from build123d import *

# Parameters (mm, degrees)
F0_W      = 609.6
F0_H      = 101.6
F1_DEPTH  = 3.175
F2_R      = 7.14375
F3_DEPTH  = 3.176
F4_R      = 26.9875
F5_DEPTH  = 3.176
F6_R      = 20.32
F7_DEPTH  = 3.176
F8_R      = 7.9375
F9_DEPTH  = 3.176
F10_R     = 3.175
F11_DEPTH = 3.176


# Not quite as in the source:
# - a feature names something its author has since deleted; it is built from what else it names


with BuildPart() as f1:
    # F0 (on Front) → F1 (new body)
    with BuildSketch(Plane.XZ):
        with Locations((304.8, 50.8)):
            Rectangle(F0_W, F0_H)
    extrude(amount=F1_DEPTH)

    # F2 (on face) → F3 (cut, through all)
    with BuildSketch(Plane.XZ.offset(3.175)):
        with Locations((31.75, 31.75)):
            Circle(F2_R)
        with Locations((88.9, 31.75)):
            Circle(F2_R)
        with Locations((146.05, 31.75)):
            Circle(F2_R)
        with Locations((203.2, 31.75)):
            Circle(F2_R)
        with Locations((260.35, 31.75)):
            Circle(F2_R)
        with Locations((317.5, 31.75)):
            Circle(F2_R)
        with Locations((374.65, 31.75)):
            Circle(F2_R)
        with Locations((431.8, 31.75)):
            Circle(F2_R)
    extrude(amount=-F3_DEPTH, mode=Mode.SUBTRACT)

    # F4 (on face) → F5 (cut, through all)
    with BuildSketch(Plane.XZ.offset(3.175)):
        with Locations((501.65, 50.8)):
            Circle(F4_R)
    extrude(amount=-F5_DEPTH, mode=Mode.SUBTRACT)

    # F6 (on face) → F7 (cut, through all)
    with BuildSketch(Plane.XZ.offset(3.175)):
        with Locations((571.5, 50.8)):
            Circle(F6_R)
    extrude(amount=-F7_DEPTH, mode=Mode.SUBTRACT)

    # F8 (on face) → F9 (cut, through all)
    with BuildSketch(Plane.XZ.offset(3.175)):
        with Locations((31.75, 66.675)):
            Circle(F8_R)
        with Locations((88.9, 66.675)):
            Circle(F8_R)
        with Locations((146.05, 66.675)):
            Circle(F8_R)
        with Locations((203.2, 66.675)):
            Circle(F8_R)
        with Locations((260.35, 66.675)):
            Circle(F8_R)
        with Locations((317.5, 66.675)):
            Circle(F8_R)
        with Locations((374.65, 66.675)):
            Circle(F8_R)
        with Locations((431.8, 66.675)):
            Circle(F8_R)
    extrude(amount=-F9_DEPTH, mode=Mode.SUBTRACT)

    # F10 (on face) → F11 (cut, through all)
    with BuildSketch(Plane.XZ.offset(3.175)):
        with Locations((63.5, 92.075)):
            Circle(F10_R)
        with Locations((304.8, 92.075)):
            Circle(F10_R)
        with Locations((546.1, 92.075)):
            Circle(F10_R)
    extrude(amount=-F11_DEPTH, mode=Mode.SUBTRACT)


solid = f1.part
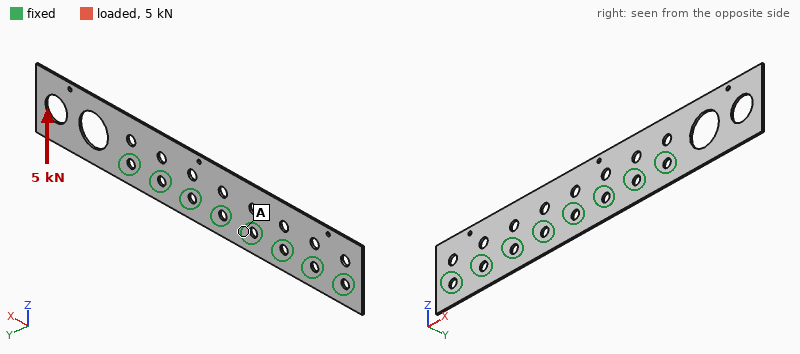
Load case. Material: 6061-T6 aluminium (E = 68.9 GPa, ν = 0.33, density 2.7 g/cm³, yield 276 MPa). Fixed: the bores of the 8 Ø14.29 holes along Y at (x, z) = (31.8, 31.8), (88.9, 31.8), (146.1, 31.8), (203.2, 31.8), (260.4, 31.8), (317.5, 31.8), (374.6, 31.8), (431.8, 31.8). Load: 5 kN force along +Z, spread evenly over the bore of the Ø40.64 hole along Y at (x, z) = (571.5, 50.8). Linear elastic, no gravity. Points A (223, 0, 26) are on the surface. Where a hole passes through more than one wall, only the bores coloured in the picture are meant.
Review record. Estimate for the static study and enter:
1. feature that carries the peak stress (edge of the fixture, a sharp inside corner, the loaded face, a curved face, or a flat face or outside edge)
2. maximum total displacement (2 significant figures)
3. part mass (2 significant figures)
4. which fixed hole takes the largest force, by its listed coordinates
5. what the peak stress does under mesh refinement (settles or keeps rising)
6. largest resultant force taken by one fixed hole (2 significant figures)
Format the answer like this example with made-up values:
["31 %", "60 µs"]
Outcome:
["edge of the fixture", "1.1 mm", "470 g", "(431.8, 31.8)", "keeps rising", "11 kN"]
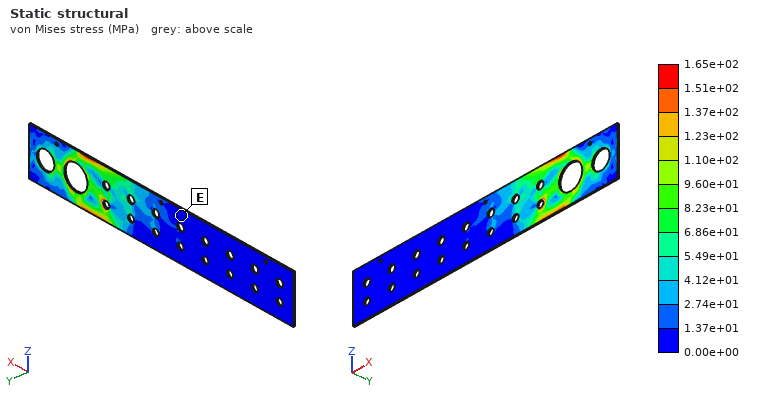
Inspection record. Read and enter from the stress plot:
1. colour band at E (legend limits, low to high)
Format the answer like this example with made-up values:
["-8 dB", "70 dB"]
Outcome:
["0.00e+00 to 1.37e+01 MPa"]
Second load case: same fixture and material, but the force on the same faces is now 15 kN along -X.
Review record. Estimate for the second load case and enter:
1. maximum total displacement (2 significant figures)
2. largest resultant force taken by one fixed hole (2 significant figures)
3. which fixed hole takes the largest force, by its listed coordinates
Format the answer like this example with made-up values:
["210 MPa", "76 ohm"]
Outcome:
["0.27 mm", "9.7 kN", "(431.8, 31.8)"]
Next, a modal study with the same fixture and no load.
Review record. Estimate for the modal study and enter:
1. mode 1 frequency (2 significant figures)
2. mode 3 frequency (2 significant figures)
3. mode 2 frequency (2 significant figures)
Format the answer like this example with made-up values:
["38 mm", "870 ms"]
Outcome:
["79 Hz", "470 Hz", "240 Hz"]
